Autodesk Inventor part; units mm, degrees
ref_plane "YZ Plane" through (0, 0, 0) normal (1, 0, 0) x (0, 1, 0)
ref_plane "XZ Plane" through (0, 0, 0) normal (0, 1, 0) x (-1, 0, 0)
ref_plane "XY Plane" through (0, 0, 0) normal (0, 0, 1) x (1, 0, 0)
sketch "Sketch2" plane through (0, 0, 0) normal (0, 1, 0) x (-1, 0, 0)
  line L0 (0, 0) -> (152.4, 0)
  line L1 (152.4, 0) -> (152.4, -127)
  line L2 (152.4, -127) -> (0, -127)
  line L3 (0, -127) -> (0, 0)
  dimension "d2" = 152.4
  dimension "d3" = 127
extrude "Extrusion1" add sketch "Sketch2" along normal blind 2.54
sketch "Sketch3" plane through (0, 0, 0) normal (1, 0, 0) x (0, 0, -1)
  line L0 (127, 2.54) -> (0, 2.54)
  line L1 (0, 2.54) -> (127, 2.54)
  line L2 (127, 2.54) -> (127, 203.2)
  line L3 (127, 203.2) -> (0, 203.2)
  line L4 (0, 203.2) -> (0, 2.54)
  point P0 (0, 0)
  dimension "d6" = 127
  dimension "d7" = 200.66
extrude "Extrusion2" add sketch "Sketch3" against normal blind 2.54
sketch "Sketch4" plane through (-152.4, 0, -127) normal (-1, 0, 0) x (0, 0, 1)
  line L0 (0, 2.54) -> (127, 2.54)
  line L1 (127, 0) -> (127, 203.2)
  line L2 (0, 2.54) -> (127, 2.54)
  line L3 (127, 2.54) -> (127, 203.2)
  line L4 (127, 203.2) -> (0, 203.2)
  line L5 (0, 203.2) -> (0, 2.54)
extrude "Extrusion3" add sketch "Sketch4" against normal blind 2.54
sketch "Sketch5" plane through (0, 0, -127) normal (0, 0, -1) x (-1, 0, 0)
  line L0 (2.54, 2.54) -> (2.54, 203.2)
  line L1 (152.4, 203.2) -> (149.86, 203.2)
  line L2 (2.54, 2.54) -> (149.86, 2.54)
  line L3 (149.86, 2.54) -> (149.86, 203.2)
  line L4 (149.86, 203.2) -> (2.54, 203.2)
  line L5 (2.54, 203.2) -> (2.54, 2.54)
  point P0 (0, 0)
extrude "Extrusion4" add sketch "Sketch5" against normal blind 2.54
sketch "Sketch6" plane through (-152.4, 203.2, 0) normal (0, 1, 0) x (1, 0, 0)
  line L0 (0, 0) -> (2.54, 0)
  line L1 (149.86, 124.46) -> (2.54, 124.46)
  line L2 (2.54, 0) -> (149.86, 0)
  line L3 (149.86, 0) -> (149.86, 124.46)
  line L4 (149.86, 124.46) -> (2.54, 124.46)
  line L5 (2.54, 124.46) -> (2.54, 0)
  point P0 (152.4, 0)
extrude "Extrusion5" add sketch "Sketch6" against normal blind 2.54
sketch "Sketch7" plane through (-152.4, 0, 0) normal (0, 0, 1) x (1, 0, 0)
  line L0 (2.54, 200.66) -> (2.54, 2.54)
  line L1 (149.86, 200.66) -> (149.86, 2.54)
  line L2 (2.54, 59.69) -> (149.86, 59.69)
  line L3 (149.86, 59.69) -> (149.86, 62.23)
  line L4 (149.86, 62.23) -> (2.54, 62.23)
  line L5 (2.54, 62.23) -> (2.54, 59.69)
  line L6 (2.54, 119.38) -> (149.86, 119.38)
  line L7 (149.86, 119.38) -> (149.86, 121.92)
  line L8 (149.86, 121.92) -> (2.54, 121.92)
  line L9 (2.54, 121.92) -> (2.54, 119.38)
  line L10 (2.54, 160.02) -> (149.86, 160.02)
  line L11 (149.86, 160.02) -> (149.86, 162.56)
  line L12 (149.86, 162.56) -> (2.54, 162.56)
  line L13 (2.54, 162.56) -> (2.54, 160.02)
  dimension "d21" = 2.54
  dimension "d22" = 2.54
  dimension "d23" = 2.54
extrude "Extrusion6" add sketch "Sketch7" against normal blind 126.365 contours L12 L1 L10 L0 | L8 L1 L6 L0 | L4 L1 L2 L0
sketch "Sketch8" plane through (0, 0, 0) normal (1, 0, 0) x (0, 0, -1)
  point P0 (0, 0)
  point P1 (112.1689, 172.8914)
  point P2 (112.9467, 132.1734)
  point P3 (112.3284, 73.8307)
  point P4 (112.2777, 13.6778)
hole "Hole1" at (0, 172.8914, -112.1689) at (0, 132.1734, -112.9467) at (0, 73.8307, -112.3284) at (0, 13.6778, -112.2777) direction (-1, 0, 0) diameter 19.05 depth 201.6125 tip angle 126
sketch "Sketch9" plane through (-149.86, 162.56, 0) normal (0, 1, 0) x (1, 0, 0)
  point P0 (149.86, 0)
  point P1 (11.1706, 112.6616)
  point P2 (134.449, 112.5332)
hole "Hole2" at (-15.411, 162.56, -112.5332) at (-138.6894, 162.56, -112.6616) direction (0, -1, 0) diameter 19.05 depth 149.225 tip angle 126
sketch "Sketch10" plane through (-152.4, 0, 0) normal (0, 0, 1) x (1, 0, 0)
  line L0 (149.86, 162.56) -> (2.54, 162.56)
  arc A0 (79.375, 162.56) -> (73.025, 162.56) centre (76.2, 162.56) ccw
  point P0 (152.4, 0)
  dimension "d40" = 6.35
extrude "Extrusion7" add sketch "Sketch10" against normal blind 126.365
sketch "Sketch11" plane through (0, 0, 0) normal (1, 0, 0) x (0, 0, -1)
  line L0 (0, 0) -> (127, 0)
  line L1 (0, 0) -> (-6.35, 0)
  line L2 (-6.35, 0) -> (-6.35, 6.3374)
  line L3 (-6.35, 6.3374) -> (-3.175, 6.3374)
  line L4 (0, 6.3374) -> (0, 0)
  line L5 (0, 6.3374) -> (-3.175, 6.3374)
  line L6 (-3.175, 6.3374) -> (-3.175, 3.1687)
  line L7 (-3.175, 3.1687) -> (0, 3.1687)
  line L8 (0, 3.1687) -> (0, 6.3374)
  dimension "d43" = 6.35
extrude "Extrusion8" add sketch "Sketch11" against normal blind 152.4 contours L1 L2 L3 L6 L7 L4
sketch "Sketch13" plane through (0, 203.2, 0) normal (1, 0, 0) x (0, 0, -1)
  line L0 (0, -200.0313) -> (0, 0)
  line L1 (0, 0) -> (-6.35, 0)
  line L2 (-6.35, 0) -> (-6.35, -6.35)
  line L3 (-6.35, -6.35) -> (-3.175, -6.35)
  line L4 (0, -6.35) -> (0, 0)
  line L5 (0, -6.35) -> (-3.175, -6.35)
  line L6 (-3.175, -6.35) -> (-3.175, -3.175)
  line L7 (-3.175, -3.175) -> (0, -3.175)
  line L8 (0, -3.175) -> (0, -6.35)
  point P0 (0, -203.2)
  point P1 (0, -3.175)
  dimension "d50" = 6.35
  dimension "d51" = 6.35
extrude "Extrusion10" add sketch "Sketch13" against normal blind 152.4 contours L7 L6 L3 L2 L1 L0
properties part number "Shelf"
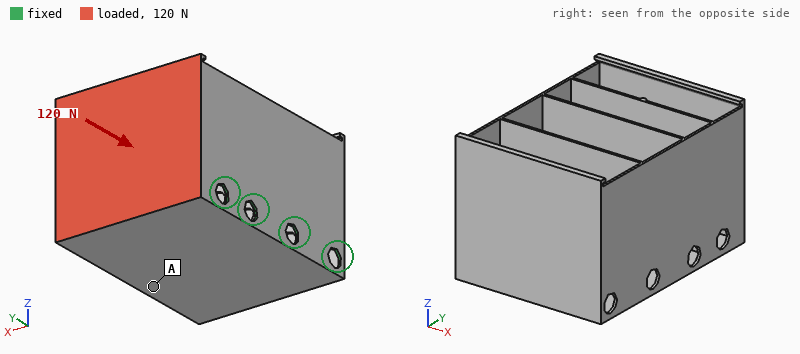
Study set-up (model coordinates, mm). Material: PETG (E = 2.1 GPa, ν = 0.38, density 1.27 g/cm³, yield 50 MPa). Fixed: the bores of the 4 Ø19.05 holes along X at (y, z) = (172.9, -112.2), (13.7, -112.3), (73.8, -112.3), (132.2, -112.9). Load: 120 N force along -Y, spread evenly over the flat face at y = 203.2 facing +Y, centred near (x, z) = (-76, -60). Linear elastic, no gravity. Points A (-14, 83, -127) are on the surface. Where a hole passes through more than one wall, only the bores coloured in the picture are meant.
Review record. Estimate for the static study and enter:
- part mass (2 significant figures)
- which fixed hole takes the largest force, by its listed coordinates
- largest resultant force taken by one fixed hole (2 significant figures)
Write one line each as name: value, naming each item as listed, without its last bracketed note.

part mass: 560 g
which fixed hole takes the largest force, by its listed coordinates: (13.7, -112.3)
largest resultant force taken by one fixed hole: 70 N
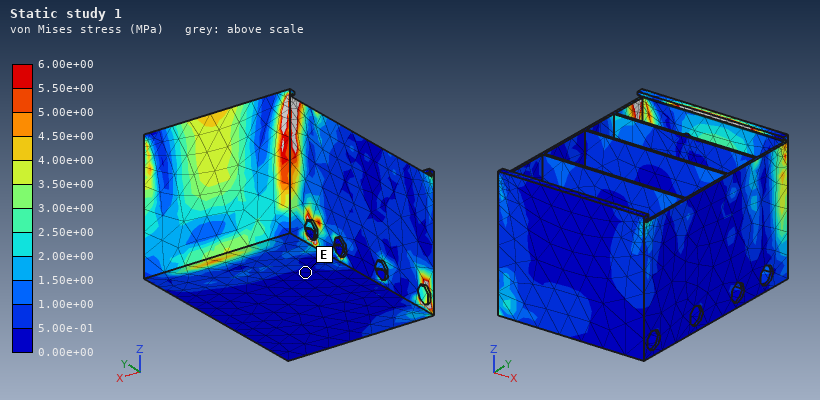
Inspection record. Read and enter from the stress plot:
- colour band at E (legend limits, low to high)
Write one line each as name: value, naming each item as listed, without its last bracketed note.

colour band at E: 0.00e+00 to 5.00e-01 MPa
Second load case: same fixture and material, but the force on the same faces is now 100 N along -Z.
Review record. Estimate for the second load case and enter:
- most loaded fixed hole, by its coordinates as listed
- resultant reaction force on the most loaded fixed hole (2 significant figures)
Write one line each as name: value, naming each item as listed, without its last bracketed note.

most loaded fixed hole, by its coordinates as listed: (172.9, -112.2)
resultant reaction force on the most loaded fixed hole: 100 N
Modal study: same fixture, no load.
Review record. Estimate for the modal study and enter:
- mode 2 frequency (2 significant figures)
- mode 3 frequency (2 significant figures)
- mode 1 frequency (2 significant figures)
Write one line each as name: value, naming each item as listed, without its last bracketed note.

mode 2 frequency: 71 Hz
mode 3 frequency: 150 Hz
mode 1 frequency: 61 Hz
